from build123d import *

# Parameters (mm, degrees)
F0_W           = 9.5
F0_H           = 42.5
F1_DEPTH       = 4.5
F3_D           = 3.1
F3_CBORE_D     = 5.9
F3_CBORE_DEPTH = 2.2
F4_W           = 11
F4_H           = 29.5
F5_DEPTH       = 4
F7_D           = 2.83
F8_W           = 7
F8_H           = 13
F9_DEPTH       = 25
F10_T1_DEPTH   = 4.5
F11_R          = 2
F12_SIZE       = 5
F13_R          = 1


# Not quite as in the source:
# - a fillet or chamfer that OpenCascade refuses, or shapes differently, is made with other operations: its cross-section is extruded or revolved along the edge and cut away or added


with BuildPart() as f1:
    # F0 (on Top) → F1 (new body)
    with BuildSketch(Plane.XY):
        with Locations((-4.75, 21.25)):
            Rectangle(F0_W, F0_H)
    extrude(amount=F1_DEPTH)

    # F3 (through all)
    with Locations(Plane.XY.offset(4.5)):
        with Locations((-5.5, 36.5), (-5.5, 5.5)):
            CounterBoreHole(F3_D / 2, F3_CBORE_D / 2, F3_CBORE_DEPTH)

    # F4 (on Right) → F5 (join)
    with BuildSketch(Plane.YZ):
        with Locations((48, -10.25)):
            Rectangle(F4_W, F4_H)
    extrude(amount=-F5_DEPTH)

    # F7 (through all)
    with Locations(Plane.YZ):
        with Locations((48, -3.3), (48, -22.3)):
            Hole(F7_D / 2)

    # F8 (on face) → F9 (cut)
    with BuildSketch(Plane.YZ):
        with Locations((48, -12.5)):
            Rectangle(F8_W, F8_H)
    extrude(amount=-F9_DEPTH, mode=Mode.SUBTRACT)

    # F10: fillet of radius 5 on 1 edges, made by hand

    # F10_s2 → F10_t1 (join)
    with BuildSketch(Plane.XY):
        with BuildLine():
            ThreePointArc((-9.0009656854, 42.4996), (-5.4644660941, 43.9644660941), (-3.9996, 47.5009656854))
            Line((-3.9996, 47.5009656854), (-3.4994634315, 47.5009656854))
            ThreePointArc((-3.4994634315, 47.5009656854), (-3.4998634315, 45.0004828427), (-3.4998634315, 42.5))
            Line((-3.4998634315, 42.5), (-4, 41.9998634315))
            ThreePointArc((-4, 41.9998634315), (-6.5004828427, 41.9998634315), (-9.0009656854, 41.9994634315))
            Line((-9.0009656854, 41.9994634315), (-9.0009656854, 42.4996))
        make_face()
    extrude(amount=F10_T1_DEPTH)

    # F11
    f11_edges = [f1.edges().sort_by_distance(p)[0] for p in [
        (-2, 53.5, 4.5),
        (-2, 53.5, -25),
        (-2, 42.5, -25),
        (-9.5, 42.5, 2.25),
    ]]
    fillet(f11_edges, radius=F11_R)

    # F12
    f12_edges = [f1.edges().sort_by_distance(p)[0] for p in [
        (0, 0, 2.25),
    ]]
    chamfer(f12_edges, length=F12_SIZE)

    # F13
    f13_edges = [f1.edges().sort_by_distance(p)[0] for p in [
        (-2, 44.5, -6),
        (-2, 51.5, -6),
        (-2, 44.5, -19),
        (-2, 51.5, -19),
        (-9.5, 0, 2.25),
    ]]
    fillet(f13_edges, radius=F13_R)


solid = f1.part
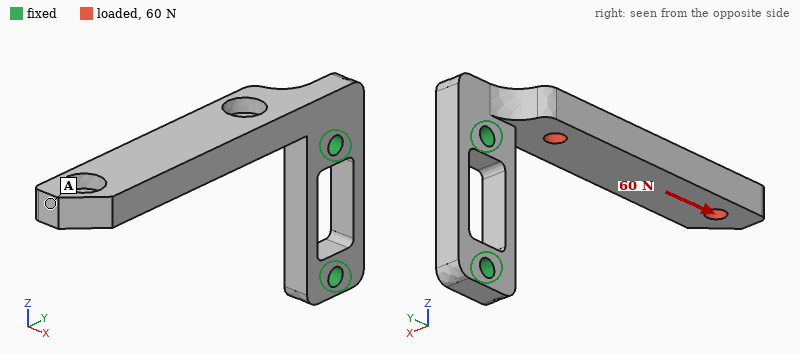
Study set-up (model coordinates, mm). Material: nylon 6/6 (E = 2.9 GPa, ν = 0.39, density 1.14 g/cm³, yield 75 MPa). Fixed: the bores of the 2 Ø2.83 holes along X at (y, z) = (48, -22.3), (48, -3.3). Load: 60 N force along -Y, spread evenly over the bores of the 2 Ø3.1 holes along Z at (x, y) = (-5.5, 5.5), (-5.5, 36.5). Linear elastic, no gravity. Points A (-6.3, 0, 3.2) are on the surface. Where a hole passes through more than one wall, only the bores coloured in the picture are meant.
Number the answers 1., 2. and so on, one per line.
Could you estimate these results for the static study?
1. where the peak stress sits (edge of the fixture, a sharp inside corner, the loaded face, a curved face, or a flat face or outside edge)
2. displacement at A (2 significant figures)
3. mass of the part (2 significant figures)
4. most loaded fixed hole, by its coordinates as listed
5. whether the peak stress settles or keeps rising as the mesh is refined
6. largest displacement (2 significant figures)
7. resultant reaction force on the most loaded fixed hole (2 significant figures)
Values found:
1. edge of the fixture
2. 0.60 mm
3. 2.9 g
4. (48, -3.3)
5. keeps rising
6. 0.61 mm
7. 61 N
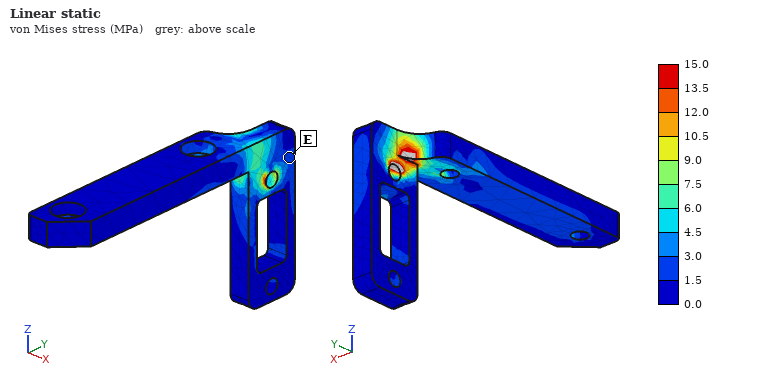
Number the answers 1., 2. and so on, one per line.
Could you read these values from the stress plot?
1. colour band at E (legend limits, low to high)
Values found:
1. 1.5 to 3.0 MPa
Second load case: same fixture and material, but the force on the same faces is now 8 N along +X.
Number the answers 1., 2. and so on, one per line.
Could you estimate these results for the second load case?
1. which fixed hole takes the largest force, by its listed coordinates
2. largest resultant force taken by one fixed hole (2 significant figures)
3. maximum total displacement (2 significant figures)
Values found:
1. (48, -3.3)
2. 8.3 N
3. 0.64 mm
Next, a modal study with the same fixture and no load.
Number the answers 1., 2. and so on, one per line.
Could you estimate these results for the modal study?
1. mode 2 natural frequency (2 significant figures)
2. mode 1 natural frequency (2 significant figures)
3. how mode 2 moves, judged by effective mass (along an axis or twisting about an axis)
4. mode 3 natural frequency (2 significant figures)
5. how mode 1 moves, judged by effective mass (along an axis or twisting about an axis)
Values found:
1. 540 Hz
2. 470 Hz
3. along X
4. 2900 Hz
5. along Z
